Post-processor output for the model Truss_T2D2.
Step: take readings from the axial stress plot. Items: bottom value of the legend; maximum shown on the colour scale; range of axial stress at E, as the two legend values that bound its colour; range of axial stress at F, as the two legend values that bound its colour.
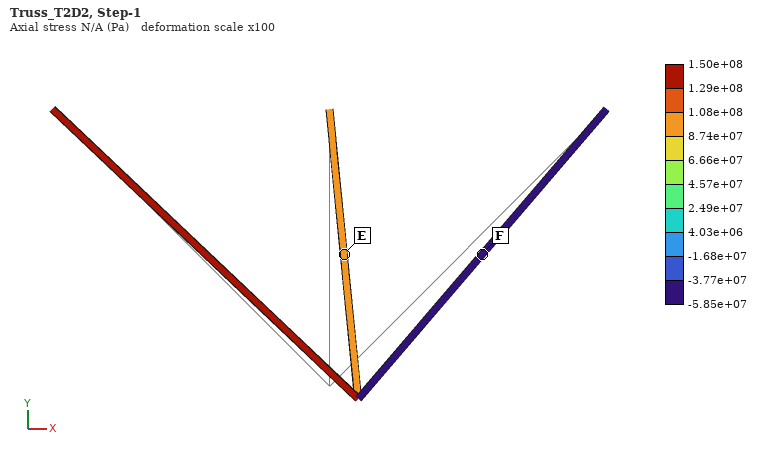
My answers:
-5.85e+07 Pa
1.50e+08 Pa
8.74e+07 to 1.08e+08 Pa
-5.85e+07 to -3.77e+07 Pa
